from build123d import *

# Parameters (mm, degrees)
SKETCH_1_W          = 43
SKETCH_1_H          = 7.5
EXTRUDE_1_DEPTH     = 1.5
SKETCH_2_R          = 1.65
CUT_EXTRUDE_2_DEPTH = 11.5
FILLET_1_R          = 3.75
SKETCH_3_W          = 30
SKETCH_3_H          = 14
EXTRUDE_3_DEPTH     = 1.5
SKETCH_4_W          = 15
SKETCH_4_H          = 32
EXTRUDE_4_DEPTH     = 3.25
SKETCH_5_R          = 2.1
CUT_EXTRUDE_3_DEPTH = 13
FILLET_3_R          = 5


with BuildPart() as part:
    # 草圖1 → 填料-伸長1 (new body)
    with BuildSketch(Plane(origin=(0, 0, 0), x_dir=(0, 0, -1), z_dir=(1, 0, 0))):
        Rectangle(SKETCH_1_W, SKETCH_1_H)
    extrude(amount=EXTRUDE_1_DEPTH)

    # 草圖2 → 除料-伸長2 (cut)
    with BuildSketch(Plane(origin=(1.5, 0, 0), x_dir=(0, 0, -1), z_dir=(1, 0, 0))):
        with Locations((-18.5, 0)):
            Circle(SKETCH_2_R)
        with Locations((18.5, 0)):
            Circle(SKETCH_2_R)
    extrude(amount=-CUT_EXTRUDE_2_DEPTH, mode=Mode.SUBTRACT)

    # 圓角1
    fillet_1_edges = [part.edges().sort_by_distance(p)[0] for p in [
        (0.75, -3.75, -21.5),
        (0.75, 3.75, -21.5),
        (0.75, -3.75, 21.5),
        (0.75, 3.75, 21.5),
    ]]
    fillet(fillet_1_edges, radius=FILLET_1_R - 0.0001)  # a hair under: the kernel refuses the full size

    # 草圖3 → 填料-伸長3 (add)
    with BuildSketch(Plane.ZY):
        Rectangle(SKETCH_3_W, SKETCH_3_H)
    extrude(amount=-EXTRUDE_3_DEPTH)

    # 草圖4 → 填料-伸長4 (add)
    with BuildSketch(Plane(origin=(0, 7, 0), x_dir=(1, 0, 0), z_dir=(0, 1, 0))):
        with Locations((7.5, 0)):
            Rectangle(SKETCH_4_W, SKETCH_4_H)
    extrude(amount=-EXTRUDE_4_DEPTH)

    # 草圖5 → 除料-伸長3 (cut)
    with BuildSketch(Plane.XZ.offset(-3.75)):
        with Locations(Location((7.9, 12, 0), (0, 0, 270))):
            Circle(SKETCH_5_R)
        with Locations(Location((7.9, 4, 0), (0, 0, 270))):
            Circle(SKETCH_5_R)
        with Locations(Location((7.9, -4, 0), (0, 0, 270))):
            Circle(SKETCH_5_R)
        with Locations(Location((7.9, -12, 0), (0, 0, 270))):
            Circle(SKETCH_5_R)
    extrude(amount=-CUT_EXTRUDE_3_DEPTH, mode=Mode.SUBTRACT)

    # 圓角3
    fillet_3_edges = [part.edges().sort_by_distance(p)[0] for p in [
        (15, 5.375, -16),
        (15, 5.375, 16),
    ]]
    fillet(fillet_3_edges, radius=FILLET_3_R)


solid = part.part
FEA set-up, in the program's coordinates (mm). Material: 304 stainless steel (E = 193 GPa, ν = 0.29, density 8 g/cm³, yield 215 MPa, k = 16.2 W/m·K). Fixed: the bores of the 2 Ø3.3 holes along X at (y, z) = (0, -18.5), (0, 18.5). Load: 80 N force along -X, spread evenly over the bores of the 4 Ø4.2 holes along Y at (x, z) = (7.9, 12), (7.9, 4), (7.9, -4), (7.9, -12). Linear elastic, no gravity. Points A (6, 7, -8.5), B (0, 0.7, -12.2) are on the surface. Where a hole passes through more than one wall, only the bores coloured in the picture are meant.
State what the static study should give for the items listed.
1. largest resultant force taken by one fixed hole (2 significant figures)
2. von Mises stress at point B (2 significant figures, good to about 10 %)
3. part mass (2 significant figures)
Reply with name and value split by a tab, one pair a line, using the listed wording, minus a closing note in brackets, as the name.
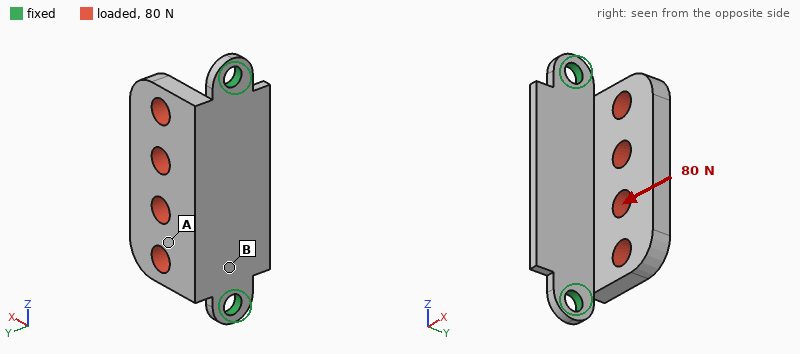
largest resultant force taken by one fixed hole	43 N
von Mises stress at point B	15 MPa
part mass	15 g
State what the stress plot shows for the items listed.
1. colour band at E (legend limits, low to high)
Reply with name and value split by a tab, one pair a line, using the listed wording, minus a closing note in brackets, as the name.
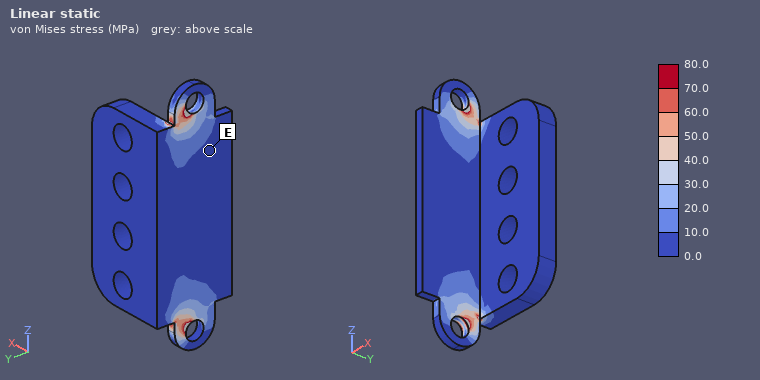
colour band at E	0.0 to 10.0 MPa
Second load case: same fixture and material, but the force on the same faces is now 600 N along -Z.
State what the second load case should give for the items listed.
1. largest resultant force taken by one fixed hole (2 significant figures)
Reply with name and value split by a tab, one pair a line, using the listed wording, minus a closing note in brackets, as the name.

largest resultant force taken by one fixed hole	340 N
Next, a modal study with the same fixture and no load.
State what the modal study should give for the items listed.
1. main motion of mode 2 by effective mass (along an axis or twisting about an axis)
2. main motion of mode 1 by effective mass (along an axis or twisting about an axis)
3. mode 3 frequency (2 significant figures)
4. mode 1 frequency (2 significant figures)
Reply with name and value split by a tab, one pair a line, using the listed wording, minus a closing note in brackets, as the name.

main motion of mode 2 by effective mass	along X
main motion of mode 1 by effective mass	along Y
mode 3 frequency	9500 Hz
mode 1 frequency	2500 Hz
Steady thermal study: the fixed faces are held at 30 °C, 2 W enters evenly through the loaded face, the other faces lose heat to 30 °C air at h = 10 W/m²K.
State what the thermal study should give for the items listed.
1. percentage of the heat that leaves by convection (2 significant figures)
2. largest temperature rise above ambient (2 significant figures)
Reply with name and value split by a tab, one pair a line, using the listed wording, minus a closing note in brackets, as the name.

percentage of the heat that leaves by convection	24 %
largest temperature rise above ambient	37 K
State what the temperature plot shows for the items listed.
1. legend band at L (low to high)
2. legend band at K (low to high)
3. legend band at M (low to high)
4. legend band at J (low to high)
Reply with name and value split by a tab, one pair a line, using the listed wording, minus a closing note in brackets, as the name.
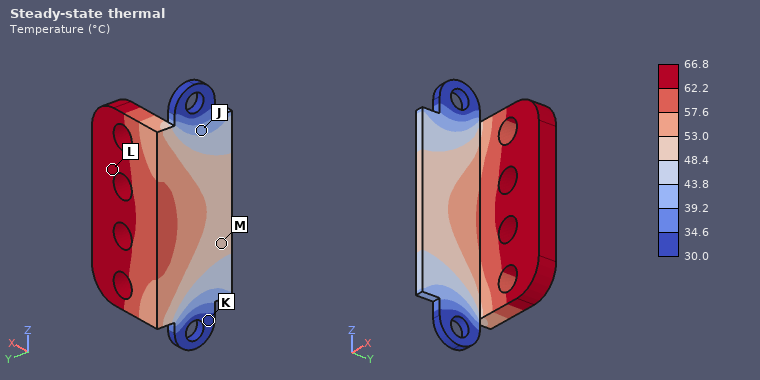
legend band at L	62.2 to 66.8 °C
legend band at K	30.0 to 34.6 °C
legend band at M	48.4 to 53.0 °C
legend band at J	39.2 to 43.8 °C
